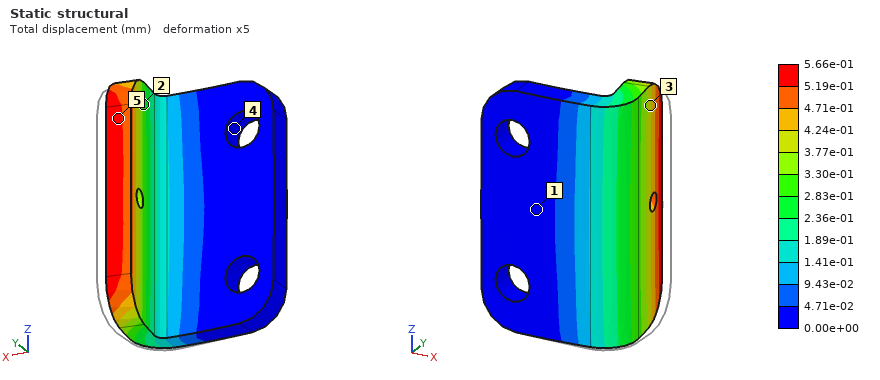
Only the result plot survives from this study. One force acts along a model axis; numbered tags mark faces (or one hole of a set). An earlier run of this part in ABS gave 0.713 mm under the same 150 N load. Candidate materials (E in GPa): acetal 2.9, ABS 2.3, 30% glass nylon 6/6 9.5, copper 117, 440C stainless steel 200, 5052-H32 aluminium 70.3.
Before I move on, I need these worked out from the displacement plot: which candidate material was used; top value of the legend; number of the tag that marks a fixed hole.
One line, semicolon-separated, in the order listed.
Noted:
acetal; 5.66e-01 mm; 4
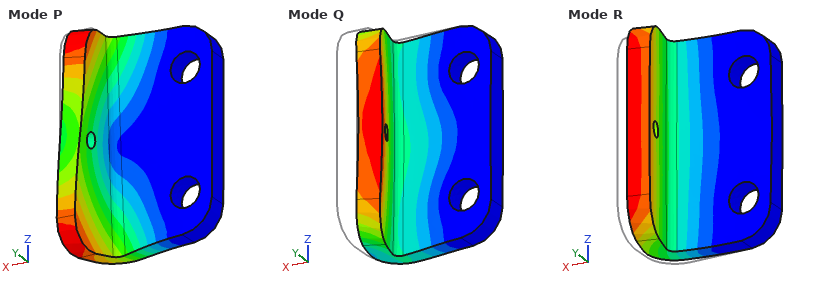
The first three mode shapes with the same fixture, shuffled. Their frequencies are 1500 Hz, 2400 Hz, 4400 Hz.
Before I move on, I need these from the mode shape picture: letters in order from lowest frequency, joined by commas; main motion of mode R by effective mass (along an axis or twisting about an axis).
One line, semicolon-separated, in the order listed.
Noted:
R, P, Q; along Y
